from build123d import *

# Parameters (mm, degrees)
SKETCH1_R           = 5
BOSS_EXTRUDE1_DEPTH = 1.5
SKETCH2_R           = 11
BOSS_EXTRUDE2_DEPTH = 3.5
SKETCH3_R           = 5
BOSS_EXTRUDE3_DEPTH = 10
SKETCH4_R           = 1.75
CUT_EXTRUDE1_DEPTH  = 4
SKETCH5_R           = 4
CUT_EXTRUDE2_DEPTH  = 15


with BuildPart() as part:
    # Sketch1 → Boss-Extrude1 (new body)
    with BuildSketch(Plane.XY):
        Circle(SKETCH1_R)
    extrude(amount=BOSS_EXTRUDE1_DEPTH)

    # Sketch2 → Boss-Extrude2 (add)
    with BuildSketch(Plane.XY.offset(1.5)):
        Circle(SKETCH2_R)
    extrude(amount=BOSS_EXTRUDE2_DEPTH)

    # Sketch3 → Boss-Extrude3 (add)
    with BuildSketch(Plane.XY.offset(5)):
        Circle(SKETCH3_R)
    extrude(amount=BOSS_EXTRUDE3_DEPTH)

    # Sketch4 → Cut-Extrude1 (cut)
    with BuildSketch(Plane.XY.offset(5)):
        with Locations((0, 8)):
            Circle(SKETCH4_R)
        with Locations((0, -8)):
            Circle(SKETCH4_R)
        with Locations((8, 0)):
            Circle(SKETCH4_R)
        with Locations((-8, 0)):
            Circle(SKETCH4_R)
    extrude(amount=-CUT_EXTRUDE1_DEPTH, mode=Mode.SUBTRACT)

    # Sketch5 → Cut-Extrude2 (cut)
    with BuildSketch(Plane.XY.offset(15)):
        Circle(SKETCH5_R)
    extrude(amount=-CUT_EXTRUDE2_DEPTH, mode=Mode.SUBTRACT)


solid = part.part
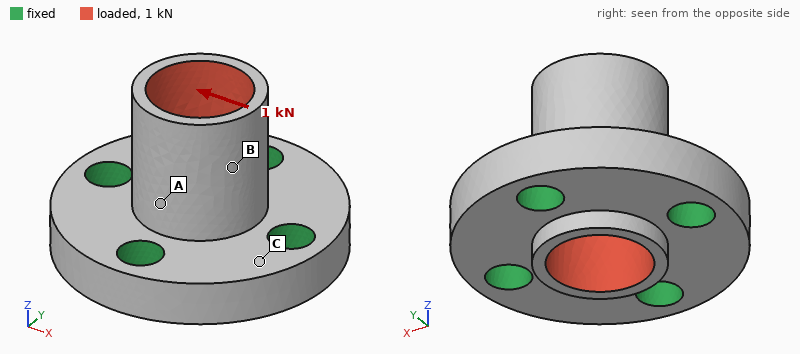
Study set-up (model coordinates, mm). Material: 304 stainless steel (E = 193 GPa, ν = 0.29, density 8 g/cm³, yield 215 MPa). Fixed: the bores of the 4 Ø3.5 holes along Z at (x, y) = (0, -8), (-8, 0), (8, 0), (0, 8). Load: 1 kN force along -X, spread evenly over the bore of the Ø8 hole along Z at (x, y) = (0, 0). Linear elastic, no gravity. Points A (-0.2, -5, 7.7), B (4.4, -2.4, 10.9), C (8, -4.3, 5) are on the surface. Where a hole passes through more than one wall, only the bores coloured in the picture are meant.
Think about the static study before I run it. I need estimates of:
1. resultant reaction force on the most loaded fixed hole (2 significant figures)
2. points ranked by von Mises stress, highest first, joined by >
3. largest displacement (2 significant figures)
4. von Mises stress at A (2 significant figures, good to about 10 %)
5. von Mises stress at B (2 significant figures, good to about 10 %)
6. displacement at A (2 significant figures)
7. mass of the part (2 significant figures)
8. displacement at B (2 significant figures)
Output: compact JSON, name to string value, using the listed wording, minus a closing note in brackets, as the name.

{"resultant reaction force on the most loaded fixed hole": "420 N", "points ranked by von Mises stress, highest first, joined by >": "A > B > C", "largest displacement": "6.9 µm", "von Mises stress at A": "47 MPa", "von Mises stress at B": "20 MPa", "displacement at A": "2.3 µm", "mass of the part": "11 g", "displacement at B": "4.9 µm"}
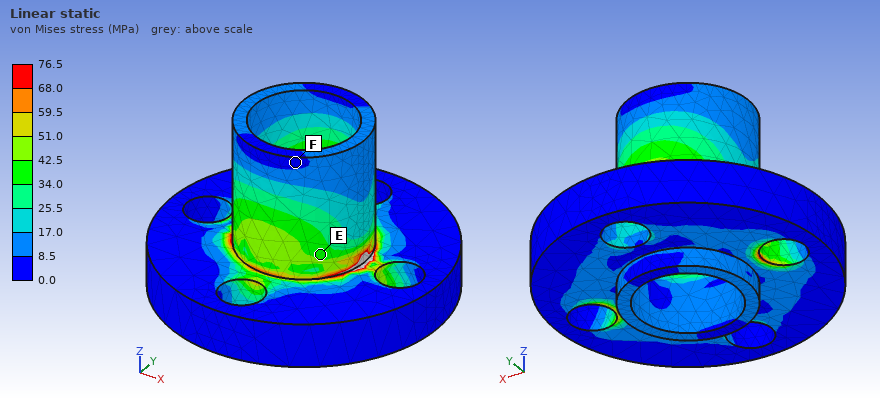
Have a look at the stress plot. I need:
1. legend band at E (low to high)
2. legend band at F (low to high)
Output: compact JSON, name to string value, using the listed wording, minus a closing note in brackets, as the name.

{"legend band at E": "34.0 to 42.5 MPa", "legend band at F": "0.0 to 8.5 MPa"}
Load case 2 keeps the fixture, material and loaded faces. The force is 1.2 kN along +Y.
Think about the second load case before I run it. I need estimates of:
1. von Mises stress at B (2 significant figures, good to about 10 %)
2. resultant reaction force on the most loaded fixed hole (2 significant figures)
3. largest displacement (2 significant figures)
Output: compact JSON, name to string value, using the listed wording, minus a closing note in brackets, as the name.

{"von Mises stress at B": "34 MPa", "resultant reaction force on the most loaded fixed hole": "500 N", "largest displacement": "8.3 µm"}
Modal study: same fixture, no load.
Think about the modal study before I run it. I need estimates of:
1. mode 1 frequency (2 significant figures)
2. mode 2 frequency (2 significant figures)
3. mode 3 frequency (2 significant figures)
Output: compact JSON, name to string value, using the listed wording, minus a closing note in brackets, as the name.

{"mode 1 frequency": "38 kHz", "mode 2 frequency": "38 kHz", "mode 3 frequency": "38 kHz"}
